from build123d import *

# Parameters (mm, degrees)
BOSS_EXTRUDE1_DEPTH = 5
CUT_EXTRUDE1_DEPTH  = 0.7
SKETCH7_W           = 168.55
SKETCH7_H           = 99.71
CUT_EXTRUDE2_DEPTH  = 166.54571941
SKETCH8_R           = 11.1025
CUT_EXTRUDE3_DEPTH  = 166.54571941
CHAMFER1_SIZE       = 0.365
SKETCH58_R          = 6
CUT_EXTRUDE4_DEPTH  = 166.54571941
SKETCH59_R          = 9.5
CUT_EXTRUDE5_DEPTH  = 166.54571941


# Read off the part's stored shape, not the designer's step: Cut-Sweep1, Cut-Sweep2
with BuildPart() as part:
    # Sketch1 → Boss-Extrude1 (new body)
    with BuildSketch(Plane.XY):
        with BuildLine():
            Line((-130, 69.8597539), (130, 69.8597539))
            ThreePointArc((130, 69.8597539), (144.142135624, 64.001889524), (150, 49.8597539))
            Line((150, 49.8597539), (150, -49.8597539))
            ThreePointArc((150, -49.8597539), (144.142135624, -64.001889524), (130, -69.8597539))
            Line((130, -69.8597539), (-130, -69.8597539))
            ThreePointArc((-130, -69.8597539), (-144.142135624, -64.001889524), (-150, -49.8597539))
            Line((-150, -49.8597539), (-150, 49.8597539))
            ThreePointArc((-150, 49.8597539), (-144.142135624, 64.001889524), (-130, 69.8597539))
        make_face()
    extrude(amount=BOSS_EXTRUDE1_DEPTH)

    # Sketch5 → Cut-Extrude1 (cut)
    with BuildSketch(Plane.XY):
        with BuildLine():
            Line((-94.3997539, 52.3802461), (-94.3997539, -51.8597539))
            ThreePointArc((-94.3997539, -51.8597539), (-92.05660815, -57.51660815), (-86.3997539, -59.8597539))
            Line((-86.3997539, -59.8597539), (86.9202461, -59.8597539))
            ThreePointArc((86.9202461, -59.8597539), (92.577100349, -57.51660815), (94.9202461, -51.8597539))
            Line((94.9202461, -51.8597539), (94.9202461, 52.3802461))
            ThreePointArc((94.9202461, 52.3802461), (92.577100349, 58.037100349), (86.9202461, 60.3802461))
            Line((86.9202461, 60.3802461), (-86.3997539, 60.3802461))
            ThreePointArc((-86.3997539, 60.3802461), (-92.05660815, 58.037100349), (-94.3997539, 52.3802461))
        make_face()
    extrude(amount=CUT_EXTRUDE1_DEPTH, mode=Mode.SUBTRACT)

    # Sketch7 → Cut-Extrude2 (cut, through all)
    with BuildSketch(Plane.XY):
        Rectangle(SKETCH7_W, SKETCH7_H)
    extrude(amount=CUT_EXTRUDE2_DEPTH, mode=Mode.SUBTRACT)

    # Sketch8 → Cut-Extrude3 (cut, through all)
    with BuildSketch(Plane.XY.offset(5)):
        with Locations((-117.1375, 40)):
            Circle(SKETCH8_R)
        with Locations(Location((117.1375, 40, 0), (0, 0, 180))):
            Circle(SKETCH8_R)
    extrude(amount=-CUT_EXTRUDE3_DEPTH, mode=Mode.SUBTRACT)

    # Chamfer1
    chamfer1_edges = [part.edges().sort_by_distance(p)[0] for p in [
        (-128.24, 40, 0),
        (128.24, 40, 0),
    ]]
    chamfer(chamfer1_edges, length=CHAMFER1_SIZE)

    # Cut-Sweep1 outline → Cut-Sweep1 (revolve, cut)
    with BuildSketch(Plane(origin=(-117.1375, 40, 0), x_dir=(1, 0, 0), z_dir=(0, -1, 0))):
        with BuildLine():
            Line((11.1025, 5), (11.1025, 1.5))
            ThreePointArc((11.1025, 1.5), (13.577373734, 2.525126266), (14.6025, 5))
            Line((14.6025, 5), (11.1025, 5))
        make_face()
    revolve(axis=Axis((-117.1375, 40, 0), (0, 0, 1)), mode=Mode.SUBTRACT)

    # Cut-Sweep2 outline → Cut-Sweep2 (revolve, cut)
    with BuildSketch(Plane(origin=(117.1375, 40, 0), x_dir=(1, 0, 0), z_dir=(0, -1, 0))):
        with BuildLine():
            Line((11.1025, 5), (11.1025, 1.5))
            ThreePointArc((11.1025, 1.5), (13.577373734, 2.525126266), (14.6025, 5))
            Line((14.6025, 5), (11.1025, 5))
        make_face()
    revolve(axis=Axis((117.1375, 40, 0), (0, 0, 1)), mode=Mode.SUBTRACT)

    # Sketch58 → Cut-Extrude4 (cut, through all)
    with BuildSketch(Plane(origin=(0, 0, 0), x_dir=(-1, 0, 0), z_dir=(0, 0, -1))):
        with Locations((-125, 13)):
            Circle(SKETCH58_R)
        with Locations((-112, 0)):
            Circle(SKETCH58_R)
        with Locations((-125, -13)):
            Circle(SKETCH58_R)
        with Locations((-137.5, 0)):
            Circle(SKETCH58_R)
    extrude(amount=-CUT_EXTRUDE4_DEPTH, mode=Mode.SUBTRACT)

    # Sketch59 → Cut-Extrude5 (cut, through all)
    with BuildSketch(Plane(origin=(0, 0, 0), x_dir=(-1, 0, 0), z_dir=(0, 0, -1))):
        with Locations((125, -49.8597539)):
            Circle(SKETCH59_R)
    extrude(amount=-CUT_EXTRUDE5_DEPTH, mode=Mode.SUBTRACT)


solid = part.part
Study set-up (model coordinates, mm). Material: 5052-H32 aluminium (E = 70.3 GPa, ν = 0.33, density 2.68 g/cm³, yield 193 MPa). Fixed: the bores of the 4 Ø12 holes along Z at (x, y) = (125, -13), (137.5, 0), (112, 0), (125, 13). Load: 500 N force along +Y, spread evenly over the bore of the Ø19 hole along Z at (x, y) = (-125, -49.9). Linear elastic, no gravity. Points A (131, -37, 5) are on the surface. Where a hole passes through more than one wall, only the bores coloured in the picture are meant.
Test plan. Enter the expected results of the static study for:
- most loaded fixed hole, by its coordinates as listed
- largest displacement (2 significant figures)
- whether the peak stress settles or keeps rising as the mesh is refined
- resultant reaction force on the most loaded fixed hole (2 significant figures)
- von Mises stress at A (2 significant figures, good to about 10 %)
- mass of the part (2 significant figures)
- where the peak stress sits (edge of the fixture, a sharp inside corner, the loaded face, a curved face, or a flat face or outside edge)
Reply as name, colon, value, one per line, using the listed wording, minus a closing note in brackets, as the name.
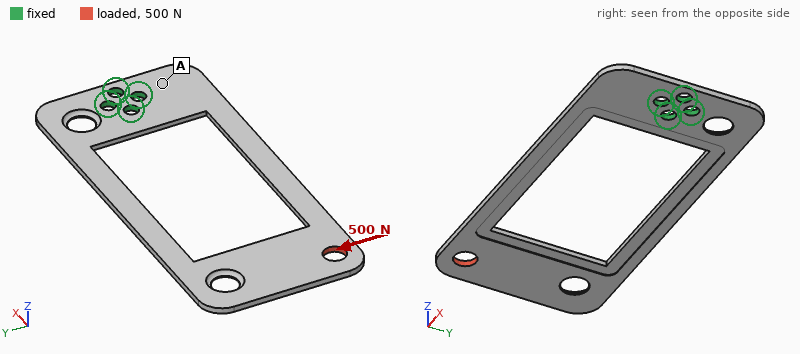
most loaded fixed hole, by its coordinates as listed: (112, 0)
largest displacement: 0.90 mm
whether the peak stress settles or keeps rising as the mesh is refined: keeps rising
resultant reaction force on the most loaded fixed hole: 2.4 kN
von Mises stress at A: 9.6 MPa
mass of the part: 300 g
where the peak stress sits: a sharp inside corner
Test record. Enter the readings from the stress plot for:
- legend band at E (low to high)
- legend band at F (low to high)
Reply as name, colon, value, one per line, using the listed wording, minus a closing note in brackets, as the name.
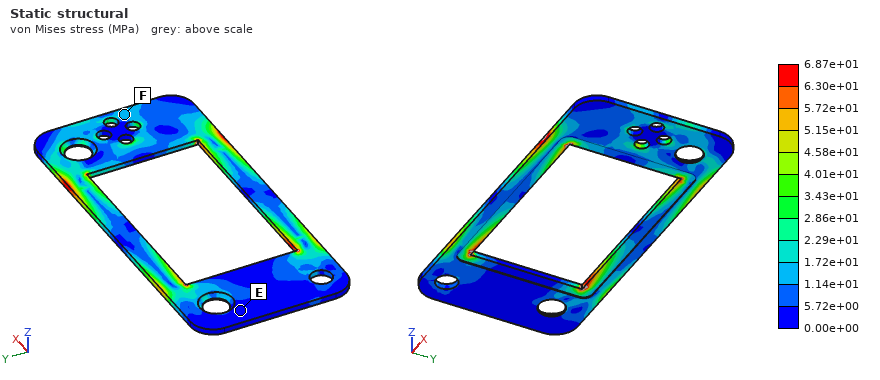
legend band at E: 0.00e+00 to 5.72e+00 MPa
legend band at F: 1.14e+01 to 1.72e+01 MPa
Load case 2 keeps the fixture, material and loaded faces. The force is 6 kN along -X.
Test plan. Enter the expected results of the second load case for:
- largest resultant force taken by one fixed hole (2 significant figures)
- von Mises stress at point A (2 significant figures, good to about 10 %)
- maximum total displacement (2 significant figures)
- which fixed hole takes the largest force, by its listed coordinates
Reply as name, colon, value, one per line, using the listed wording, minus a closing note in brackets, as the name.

largest resultant force taken by one fixed hole: 7.1 kN
von Mises stress at point A: 42 MPa
maximum total displacement: 1.4 mm
which fixed hole takes the largest force, by its listed coordinates: (125, -13)
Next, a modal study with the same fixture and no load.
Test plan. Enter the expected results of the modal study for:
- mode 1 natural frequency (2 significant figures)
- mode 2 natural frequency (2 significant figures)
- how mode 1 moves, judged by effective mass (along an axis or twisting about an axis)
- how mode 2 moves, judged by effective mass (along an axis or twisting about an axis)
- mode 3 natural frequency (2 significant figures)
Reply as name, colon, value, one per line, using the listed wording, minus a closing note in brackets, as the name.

mode 1 natural frequency: 36 Hz
mode 2 natural frequency: 140 Hz
how mode 1 moves, judged by effective mass: along Z
how mode 2 moves, judged by effective mass: twisting about X
mode 3 natural frequency: 300 Hz
